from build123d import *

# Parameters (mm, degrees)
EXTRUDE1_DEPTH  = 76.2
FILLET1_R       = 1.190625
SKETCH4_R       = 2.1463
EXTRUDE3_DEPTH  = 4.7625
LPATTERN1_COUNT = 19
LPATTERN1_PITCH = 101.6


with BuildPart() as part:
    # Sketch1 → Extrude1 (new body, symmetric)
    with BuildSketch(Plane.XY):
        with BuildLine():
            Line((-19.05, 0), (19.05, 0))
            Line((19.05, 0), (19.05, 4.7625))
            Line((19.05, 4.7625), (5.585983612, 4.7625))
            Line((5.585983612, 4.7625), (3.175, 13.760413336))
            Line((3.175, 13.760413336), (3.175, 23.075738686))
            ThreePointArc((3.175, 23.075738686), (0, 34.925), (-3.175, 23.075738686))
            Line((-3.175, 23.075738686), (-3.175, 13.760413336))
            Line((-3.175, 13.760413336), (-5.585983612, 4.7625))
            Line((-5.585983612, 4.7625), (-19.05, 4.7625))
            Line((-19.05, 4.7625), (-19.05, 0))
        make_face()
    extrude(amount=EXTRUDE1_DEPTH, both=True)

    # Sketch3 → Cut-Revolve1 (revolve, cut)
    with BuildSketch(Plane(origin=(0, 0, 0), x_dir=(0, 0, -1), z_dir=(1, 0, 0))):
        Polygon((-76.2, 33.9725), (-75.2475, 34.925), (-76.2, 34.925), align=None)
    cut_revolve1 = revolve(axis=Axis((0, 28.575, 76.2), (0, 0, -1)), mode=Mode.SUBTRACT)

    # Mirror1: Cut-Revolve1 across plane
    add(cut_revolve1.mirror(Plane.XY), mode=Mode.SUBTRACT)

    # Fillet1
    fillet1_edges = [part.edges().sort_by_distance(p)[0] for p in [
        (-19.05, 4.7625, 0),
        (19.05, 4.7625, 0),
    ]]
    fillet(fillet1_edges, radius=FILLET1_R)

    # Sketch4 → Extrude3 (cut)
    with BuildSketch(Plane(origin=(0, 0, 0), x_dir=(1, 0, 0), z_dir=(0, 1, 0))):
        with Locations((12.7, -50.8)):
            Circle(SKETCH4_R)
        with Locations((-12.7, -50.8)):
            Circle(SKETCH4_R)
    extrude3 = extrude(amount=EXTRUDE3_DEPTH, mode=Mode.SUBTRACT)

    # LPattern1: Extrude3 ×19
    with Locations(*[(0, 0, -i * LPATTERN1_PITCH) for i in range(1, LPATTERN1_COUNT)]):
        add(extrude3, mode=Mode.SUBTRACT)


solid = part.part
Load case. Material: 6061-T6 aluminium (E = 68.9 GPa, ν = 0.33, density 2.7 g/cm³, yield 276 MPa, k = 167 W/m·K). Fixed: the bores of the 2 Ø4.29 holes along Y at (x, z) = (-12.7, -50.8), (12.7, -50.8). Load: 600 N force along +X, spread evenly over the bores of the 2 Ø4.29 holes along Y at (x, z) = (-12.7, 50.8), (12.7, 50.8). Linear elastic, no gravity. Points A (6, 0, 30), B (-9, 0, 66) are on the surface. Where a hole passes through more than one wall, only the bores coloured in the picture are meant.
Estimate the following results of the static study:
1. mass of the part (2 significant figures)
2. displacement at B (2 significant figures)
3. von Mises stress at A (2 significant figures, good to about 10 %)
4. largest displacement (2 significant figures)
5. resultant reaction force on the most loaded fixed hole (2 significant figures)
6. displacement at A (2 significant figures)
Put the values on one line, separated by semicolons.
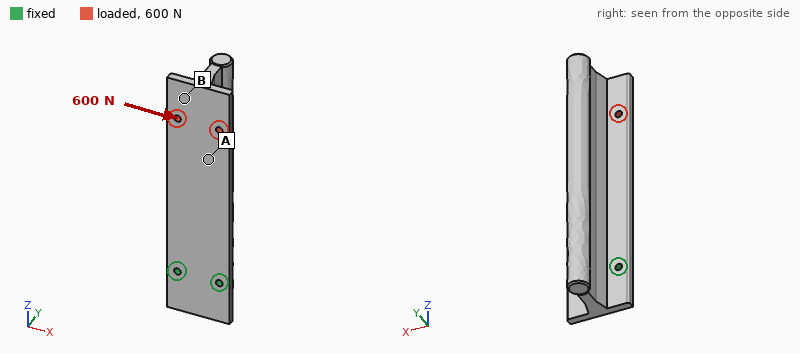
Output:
180 g; 0.18 mm; 9.4 MPa; 0.20 mm; 2.3 kN; 0.11 mm
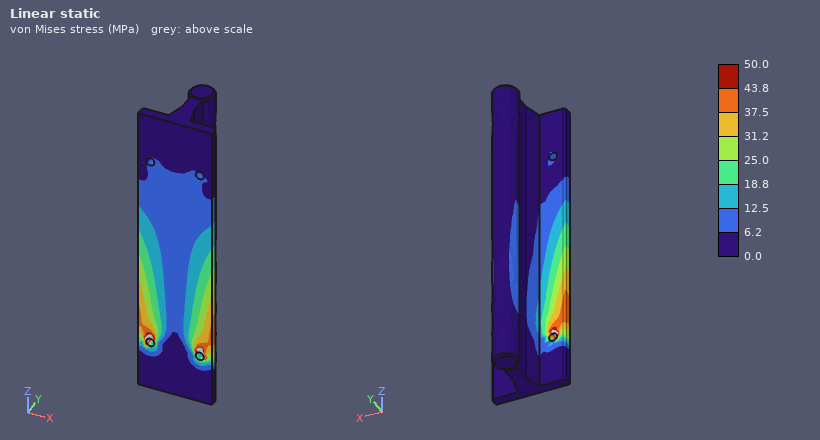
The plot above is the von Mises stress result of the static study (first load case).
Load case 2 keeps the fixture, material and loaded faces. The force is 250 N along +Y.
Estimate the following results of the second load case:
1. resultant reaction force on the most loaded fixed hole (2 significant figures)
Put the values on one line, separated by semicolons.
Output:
150 N
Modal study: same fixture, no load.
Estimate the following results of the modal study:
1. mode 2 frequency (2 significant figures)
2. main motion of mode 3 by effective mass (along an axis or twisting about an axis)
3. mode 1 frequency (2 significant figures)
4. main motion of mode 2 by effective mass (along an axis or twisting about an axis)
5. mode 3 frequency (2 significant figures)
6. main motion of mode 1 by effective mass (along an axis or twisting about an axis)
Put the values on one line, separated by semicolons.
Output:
1100 Hz; twisting about Z; 440 Hz; along X; 2000 Hz; along Y
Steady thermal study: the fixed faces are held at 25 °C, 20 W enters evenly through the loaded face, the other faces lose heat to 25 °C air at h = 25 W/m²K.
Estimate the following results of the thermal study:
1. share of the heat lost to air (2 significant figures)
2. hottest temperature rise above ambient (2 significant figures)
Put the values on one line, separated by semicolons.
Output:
36 %; 28 K
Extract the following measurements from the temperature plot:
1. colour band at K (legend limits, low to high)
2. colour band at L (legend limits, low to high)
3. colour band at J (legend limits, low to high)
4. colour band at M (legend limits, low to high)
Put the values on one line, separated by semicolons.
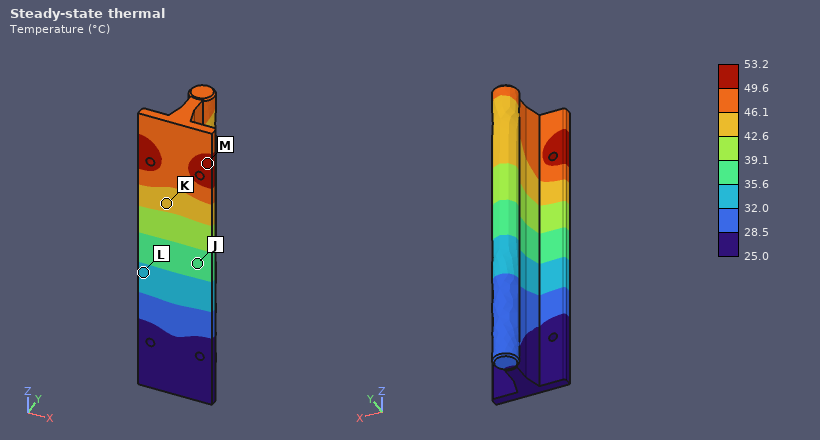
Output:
42.6 to 46.1 °C; 32.0 to 35.6 °C; 35.6 to 39.1 °C; 49.6 to 53.2 °C
